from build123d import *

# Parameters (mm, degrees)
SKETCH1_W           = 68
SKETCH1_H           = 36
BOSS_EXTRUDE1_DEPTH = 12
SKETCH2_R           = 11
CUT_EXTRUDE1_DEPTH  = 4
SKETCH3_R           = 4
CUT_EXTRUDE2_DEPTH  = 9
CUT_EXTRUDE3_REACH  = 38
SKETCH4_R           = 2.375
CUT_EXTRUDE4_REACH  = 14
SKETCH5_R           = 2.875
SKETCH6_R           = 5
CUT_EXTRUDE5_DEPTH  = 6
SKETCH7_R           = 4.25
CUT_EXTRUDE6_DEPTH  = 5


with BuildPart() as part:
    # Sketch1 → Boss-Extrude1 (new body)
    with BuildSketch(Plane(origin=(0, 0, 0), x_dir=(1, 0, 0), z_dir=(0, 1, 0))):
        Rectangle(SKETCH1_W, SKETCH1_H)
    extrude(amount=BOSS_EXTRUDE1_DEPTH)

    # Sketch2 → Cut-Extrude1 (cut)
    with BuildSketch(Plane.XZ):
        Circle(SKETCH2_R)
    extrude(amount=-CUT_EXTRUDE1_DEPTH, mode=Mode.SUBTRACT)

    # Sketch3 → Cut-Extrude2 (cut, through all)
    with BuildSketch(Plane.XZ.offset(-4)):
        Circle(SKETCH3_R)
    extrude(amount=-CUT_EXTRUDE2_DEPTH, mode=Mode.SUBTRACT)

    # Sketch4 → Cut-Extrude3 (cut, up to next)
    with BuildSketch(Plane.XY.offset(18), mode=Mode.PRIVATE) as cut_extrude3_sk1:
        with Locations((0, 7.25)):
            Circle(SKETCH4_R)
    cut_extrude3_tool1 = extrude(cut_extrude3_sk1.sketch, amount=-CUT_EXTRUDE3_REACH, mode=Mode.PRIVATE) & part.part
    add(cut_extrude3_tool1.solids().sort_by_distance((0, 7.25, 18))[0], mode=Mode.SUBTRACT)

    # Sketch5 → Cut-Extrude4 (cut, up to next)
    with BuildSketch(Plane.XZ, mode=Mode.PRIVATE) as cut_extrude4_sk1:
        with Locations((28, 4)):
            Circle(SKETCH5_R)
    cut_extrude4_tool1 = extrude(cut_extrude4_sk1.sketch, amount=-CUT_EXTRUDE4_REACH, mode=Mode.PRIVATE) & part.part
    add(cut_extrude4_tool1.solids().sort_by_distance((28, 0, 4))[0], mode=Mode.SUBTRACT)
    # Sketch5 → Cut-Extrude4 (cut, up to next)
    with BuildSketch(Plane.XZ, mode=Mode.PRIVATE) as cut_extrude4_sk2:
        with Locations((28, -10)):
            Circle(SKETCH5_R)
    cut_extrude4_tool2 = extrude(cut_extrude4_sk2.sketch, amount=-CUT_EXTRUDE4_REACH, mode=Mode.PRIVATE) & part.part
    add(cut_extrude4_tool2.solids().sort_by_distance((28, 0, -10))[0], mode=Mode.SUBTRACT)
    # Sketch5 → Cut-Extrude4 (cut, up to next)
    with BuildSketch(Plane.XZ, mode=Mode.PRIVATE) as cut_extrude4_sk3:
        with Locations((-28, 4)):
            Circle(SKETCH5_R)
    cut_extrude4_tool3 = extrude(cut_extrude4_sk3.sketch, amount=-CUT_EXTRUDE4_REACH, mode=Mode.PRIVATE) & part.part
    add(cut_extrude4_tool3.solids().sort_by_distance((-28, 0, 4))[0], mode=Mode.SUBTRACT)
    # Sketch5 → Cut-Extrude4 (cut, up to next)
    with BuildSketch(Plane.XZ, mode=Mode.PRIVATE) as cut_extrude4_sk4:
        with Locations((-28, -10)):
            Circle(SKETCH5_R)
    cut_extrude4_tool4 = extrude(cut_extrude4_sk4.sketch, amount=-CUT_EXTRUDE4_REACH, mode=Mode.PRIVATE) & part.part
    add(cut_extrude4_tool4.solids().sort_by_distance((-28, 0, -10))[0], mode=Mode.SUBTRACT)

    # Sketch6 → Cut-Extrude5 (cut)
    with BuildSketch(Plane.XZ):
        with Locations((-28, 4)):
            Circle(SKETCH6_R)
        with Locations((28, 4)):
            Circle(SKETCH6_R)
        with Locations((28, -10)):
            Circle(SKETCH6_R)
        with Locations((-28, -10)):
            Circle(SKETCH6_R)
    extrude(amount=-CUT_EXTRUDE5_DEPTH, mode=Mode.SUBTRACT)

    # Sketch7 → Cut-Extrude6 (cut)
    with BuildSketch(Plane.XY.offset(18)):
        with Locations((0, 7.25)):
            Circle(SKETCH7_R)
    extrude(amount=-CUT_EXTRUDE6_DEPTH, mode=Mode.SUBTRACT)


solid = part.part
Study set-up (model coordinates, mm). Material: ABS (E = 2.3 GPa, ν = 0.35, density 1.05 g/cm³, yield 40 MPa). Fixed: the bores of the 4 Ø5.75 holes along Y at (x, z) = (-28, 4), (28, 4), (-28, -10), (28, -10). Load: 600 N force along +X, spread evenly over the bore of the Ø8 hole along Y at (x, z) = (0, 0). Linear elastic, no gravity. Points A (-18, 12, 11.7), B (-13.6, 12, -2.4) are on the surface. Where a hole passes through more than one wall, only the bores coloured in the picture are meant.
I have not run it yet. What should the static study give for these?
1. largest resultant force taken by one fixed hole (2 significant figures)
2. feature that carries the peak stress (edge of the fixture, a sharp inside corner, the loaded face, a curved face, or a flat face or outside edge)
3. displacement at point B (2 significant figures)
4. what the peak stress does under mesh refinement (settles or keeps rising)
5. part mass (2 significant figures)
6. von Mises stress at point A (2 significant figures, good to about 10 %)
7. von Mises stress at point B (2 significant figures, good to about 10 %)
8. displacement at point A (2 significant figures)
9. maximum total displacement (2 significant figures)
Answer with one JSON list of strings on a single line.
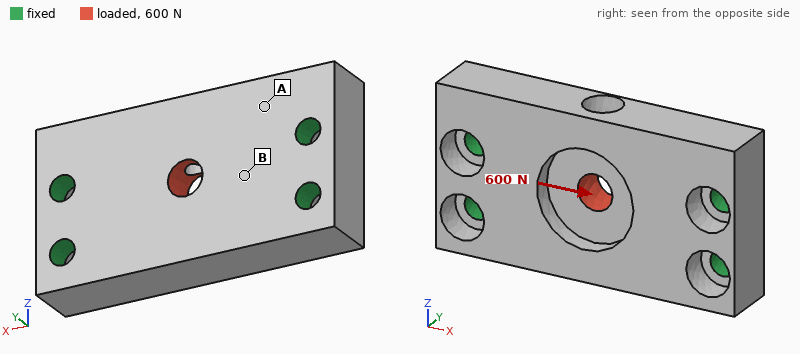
["160 N", "a sharp inside corner", "10 µm", "keeps rising", "26 g", "0.88 MPa", "2.3 MPa", "8.2 µm", "22 µm"]
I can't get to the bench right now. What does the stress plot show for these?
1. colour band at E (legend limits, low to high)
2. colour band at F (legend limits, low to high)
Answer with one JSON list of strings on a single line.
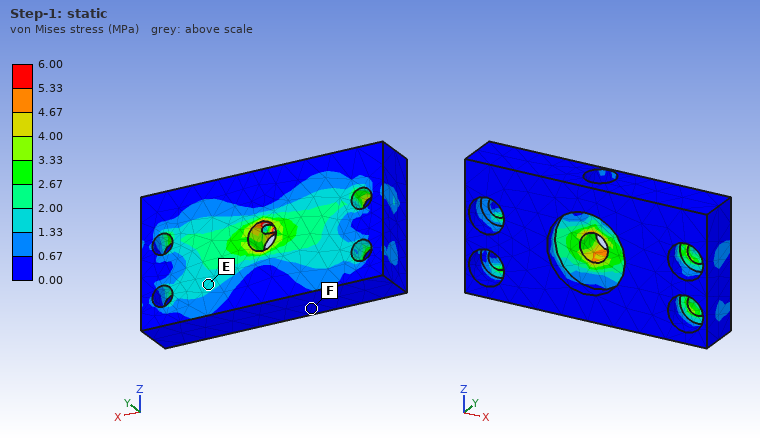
["1.33 to 2.00 MPa", "0.00 to 0.67 MPa"]
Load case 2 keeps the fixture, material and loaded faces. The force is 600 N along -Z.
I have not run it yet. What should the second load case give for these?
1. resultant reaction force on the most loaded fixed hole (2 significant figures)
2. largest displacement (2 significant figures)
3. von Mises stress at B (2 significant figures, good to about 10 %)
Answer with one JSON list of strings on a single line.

["200 N", "53 µm", "2.3 MPa"]
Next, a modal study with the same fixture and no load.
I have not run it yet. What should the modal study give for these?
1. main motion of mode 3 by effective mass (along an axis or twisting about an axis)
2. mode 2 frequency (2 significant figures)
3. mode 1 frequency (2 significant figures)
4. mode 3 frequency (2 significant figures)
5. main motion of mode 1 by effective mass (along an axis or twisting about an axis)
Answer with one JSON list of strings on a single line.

["along Z", "4200 Hz", "3400 Hz", "5900 Hz", "along Y"]
